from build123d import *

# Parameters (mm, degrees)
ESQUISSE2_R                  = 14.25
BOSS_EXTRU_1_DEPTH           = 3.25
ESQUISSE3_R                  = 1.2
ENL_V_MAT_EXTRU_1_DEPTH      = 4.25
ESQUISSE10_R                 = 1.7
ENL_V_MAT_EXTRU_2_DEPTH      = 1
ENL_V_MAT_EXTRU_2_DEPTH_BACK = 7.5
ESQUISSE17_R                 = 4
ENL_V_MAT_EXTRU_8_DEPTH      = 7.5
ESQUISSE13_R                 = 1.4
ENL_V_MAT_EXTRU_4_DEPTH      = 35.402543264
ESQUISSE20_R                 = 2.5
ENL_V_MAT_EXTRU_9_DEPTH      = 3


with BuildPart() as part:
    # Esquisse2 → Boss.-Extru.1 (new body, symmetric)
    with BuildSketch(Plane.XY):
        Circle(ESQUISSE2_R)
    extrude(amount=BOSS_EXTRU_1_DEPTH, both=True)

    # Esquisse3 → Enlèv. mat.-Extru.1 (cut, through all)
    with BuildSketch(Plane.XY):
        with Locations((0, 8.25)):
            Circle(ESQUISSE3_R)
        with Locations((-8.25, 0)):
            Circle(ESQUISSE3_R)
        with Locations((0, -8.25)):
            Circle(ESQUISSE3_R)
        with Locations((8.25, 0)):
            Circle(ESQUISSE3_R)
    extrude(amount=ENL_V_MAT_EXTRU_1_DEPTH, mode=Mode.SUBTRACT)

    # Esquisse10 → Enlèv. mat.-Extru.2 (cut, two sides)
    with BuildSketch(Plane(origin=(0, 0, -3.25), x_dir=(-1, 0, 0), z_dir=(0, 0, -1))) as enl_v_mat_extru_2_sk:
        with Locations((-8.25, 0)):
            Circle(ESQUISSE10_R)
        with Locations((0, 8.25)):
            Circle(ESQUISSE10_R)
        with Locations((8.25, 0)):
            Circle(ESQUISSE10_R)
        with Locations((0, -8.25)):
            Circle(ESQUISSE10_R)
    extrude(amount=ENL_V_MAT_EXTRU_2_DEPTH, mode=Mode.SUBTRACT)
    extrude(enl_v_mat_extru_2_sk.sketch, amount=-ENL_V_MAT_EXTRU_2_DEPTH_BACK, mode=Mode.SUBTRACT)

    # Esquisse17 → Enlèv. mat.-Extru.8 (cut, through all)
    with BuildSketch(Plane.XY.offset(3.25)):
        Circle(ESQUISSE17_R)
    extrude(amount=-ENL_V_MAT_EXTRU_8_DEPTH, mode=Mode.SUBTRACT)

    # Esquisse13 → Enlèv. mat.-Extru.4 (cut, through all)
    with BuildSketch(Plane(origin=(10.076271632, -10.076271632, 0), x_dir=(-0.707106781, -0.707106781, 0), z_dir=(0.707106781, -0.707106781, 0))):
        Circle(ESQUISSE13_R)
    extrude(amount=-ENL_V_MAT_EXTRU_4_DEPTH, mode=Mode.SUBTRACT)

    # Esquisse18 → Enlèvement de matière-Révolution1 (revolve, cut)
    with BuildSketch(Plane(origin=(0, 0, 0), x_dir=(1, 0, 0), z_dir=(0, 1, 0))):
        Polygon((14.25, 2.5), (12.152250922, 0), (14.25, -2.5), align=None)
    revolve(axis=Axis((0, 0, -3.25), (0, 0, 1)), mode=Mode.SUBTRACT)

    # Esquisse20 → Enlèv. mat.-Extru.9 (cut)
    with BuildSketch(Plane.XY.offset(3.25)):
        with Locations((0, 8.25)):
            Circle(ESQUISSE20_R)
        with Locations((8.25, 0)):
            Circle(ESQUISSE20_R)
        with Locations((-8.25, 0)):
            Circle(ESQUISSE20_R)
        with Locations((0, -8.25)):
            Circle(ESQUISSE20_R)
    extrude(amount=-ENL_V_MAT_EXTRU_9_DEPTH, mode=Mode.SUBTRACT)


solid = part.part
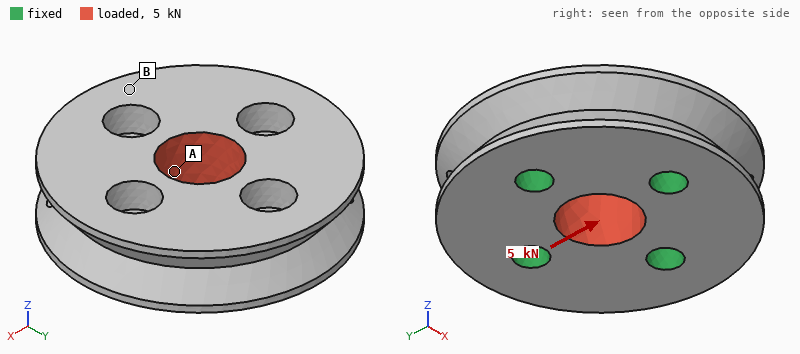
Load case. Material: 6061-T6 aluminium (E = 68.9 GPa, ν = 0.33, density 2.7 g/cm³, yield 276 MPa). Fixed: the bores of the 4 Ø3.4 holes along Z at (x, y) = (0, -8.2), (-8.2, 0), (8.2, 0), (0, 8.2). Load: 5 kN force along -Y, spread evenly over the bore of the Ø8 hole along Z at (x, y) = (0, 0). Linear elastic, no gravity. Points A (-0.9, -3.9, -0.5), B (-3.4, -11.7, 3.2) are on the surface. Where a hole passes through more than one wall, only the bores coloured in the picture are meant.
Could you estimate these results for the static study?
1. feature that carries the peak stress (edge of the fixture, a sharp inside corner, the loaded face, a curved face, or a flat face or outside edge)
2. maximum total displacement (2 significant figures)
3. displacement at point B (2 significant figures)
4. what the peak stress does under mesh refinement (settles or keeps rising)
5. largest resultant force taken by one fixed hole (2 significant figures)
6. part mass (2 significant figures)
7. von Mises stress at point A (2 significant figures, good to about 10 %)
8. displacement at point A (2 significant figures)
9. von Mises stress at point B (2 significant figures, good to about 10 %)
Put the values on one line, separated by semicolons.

edge of the fixture; 8.0 µm; 3.6 µm; keeps rising; 1.4 kN; 7.8 g; 57 MPa; 3.1 µm; 15 MPa
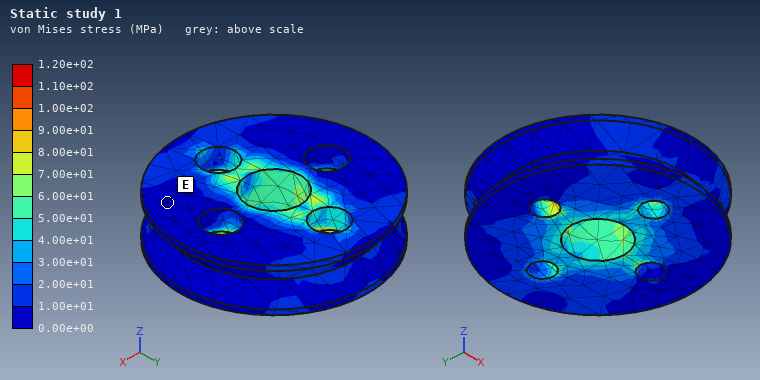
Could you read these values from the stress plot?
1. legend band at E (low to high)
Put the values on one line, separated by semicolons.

0.00e+00 to 1.00e+01 MPa
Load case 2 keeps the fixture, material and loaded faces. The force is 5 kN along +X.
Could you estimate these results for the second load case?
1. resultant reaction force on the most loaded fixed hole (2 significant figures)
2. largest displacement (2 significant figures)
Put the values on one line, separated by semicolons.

1.4 kN; 8.1 µm
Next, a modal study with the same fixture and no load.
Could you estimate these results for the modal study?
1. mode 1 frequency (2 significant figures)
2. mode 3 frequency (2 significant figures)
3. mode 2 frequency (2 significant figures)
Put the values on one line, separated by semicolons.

46 kHz; 52 kHz; 50 kHz
